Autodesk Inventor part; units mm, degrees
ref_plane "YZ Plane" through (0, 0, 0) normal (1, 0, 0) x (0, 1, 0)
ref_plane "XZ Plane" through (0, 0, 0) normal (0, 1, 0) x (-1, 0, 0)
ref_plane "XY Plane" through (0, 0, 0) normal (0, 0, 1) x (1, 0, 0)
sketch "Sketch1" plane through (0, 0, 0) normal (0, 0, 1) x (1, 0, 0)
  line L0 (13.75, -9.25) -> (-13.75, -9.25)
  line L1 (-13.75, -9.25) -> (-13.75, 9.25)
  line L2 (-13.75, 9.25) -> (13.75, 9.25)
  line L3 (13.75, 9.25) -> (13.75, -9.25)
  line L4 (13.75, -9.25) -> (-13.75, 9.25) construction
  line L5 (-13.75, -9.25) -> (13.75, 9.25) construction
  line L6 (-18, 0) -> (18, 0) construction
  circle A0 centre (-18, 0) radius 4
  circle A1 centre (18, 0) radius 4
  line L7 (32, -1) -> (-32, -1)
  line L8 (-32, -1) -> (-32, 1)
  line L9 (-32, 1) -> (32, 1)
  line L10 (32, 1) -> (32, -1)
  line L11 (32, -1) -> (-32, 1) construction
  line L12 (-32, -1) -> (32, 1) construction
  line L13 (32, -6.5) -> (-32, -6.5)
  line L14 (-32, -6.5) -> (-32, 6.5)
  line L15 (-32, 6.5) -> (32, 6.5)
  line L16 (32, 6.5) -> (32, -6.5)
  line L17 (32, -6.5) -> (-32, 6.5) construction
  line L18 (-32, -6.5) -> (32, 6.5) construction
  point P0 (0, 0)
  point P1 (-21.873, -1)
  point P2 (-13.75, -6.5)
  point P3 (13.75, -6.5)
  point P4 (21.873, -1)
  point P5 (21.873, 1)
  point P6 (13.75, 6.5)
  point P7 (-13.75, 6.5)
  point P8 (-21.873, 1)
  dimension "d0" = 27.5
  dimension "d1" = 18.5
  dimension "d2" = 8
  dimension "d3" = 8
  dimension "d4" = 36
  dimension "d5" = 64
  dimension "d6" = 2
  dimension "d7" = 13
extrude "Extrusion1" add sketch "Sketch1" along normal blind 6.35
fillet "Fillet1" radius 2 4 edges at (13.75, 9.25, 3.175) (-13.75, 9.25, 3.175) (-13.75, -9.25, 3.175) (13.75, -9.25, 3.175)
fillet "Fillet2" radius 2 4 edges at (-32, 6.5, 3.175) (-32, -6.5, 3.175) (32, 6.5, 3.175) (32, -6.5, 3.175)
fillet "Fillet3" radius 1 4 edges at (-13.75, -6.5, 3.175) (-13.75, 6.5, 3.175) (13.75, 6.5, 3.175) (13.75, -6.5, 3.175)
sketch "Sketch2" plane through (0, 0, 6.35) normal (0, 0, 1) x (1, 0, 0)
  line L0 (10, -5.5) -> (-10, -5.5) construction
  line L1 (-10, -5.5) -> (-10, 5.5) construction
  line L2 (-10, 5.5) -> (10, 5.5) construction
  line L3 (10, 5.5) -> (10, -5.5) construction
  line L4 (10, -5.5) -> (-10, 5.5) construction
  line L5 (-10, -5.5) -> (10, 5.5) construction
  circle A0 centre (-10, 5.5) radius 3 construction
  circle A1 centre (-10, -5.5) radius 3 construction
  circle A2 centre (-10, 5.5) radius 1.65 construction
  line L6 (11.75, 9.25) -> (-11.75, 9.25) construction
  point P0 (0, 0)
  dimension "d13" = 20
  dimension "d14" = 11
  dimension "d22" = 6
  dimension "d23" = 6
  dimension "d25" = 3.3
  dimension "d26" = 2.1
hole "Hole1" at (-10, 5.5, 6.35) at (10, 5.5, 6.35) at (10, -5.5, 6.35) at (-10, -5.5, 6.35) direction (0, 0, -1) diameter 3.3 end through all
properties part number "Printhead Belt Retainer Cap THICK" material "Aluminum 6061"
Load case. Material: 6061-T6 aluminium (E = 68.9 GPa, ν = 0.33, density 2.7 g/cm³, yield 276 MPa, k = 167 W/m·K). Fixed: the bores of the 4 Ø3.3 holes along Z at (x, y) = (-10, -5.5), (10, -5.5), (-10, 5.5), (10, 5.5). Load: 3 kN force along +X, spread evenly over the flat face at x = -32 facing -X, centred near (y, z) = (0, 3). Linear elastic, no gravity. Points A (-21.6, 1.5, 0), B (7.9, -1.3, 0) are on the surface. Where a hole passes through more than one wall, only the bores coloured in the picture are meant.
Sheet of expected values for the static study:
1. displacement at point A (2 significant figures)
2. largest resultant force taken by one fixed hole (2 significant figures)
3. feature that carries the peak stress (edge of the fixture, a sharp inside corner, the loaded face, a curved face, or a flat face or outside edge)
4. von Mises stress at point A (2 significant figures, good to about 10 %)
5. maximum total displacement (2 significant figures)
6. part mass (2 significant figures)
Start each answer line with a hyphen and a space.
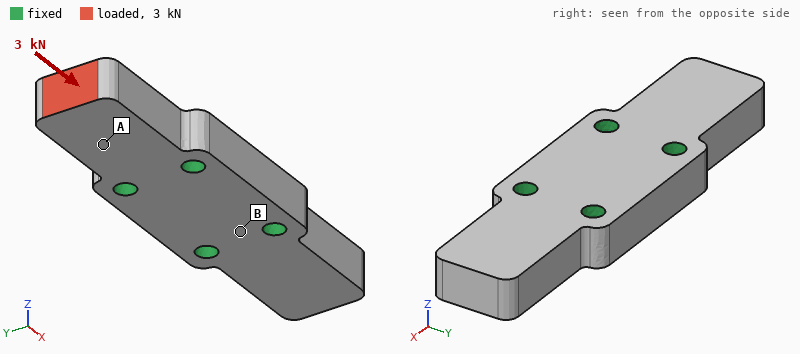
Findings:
- 5.8 µm
- 1.5 kN
- a curved face
- 38 MPa
- 13 µm
- 16 g
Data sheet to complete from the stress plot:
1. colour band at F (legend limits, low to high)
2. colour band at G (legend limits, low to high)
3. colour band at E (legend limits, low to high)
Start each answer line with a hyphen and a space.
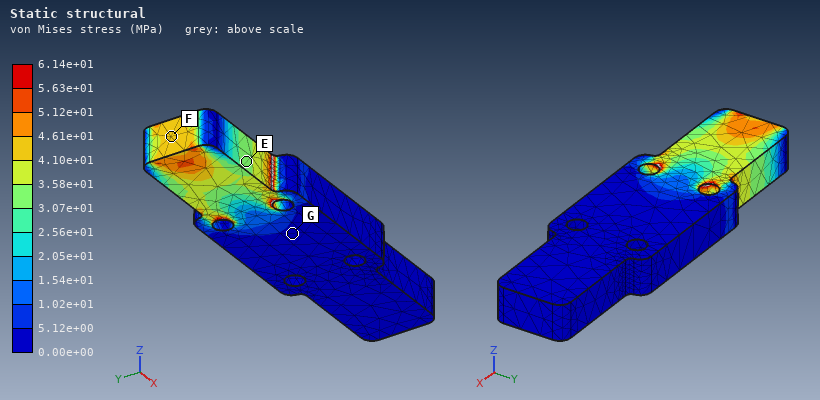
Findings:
- 4.10e+01 to 4.61e+01 MPa
- 0.00e+00 to 5.12e+00 MPa
- 3.07e+01 to 3.58e+01 MPa
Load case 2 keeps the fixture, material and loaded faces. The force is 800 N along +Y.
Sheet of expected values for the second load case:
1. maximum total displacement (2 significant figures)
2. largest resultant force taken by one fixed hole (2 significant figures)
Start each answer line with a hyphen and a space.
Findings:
- 35 µm
- 1.5 kN
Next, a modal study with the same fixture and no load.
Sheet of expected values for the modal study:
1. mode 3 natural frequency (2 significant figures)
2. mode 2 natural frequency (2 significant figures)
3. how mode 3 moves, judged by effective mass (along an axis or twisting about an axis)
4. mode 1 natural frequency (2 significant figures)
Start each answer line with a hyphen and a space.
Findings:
- 21 kHz
- 11 kHz
- along Y
- 11 kHz
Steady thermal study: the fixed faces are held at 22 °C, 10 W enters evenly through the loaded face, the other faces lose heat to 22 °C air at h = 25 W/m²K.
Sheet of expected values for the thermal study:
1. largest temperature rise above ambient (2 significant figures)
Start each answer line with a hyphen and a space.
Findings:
- 16 K
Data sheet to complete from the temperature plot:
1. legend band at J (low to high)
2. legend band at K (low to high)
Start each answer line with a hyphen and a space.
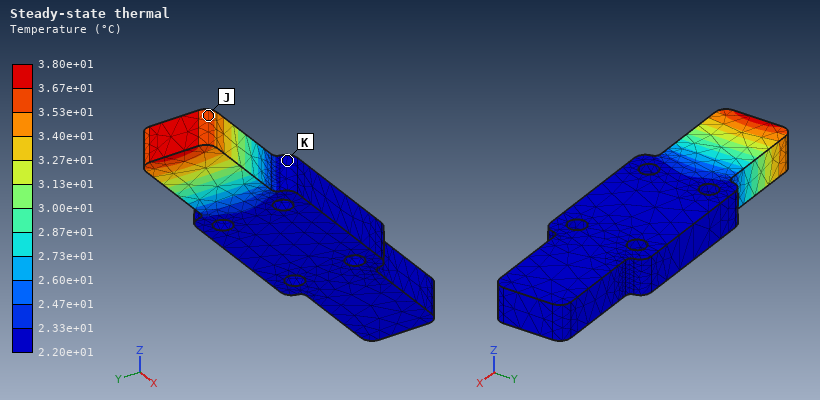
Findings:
- 3.53e+01 to 3.67e+01 °C
- 2.20e+01 to 2.33e+01 °C
